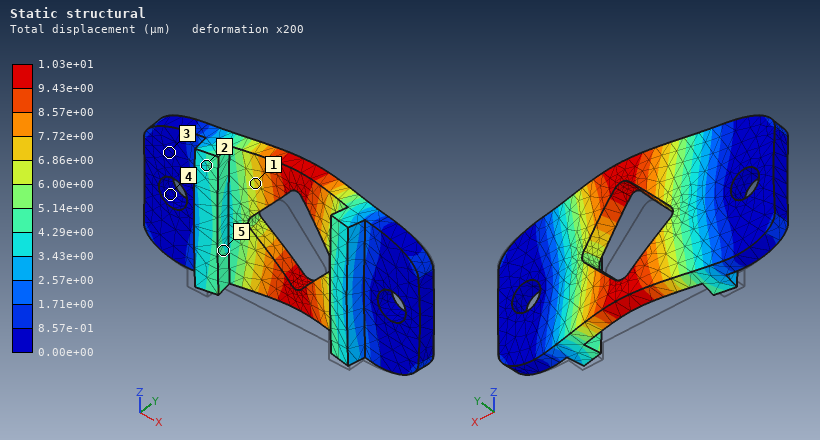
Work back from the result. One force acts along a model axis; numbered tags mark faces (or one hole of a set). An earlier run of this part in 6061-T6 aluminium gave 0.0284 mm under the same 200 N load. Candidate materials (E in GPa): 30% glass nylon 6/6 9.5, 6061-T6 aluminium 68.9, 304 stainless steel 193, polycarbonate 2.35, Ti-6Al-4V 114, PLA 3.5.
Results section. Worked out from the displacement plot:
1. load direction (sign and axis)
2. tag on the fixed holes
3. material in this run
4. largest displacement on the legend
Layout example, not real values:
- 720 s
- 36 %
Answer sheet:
- +Y
- 4
- 304 stainless steel
- 1.03e+01 µm
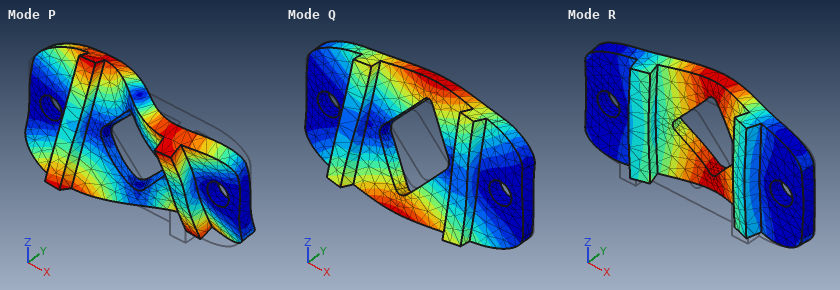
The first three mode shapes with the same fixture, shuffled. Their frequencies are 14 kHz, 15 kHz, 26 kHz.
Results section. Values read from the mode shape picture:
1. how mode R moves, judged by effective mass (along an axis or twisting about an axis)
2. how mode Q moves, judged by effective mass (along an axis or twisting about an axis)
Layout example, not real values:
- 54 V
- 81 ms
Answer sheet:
- along Y
- twisting about X
